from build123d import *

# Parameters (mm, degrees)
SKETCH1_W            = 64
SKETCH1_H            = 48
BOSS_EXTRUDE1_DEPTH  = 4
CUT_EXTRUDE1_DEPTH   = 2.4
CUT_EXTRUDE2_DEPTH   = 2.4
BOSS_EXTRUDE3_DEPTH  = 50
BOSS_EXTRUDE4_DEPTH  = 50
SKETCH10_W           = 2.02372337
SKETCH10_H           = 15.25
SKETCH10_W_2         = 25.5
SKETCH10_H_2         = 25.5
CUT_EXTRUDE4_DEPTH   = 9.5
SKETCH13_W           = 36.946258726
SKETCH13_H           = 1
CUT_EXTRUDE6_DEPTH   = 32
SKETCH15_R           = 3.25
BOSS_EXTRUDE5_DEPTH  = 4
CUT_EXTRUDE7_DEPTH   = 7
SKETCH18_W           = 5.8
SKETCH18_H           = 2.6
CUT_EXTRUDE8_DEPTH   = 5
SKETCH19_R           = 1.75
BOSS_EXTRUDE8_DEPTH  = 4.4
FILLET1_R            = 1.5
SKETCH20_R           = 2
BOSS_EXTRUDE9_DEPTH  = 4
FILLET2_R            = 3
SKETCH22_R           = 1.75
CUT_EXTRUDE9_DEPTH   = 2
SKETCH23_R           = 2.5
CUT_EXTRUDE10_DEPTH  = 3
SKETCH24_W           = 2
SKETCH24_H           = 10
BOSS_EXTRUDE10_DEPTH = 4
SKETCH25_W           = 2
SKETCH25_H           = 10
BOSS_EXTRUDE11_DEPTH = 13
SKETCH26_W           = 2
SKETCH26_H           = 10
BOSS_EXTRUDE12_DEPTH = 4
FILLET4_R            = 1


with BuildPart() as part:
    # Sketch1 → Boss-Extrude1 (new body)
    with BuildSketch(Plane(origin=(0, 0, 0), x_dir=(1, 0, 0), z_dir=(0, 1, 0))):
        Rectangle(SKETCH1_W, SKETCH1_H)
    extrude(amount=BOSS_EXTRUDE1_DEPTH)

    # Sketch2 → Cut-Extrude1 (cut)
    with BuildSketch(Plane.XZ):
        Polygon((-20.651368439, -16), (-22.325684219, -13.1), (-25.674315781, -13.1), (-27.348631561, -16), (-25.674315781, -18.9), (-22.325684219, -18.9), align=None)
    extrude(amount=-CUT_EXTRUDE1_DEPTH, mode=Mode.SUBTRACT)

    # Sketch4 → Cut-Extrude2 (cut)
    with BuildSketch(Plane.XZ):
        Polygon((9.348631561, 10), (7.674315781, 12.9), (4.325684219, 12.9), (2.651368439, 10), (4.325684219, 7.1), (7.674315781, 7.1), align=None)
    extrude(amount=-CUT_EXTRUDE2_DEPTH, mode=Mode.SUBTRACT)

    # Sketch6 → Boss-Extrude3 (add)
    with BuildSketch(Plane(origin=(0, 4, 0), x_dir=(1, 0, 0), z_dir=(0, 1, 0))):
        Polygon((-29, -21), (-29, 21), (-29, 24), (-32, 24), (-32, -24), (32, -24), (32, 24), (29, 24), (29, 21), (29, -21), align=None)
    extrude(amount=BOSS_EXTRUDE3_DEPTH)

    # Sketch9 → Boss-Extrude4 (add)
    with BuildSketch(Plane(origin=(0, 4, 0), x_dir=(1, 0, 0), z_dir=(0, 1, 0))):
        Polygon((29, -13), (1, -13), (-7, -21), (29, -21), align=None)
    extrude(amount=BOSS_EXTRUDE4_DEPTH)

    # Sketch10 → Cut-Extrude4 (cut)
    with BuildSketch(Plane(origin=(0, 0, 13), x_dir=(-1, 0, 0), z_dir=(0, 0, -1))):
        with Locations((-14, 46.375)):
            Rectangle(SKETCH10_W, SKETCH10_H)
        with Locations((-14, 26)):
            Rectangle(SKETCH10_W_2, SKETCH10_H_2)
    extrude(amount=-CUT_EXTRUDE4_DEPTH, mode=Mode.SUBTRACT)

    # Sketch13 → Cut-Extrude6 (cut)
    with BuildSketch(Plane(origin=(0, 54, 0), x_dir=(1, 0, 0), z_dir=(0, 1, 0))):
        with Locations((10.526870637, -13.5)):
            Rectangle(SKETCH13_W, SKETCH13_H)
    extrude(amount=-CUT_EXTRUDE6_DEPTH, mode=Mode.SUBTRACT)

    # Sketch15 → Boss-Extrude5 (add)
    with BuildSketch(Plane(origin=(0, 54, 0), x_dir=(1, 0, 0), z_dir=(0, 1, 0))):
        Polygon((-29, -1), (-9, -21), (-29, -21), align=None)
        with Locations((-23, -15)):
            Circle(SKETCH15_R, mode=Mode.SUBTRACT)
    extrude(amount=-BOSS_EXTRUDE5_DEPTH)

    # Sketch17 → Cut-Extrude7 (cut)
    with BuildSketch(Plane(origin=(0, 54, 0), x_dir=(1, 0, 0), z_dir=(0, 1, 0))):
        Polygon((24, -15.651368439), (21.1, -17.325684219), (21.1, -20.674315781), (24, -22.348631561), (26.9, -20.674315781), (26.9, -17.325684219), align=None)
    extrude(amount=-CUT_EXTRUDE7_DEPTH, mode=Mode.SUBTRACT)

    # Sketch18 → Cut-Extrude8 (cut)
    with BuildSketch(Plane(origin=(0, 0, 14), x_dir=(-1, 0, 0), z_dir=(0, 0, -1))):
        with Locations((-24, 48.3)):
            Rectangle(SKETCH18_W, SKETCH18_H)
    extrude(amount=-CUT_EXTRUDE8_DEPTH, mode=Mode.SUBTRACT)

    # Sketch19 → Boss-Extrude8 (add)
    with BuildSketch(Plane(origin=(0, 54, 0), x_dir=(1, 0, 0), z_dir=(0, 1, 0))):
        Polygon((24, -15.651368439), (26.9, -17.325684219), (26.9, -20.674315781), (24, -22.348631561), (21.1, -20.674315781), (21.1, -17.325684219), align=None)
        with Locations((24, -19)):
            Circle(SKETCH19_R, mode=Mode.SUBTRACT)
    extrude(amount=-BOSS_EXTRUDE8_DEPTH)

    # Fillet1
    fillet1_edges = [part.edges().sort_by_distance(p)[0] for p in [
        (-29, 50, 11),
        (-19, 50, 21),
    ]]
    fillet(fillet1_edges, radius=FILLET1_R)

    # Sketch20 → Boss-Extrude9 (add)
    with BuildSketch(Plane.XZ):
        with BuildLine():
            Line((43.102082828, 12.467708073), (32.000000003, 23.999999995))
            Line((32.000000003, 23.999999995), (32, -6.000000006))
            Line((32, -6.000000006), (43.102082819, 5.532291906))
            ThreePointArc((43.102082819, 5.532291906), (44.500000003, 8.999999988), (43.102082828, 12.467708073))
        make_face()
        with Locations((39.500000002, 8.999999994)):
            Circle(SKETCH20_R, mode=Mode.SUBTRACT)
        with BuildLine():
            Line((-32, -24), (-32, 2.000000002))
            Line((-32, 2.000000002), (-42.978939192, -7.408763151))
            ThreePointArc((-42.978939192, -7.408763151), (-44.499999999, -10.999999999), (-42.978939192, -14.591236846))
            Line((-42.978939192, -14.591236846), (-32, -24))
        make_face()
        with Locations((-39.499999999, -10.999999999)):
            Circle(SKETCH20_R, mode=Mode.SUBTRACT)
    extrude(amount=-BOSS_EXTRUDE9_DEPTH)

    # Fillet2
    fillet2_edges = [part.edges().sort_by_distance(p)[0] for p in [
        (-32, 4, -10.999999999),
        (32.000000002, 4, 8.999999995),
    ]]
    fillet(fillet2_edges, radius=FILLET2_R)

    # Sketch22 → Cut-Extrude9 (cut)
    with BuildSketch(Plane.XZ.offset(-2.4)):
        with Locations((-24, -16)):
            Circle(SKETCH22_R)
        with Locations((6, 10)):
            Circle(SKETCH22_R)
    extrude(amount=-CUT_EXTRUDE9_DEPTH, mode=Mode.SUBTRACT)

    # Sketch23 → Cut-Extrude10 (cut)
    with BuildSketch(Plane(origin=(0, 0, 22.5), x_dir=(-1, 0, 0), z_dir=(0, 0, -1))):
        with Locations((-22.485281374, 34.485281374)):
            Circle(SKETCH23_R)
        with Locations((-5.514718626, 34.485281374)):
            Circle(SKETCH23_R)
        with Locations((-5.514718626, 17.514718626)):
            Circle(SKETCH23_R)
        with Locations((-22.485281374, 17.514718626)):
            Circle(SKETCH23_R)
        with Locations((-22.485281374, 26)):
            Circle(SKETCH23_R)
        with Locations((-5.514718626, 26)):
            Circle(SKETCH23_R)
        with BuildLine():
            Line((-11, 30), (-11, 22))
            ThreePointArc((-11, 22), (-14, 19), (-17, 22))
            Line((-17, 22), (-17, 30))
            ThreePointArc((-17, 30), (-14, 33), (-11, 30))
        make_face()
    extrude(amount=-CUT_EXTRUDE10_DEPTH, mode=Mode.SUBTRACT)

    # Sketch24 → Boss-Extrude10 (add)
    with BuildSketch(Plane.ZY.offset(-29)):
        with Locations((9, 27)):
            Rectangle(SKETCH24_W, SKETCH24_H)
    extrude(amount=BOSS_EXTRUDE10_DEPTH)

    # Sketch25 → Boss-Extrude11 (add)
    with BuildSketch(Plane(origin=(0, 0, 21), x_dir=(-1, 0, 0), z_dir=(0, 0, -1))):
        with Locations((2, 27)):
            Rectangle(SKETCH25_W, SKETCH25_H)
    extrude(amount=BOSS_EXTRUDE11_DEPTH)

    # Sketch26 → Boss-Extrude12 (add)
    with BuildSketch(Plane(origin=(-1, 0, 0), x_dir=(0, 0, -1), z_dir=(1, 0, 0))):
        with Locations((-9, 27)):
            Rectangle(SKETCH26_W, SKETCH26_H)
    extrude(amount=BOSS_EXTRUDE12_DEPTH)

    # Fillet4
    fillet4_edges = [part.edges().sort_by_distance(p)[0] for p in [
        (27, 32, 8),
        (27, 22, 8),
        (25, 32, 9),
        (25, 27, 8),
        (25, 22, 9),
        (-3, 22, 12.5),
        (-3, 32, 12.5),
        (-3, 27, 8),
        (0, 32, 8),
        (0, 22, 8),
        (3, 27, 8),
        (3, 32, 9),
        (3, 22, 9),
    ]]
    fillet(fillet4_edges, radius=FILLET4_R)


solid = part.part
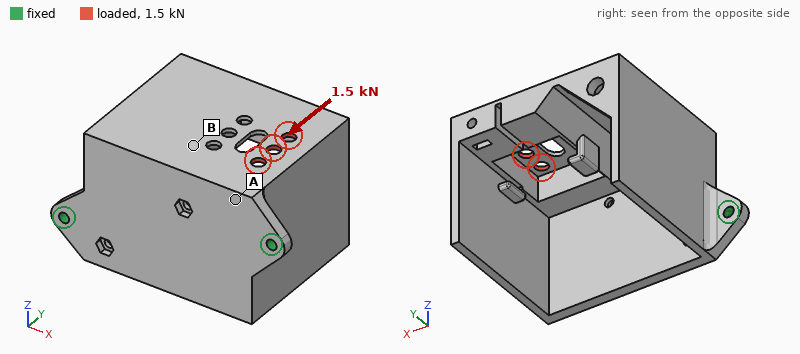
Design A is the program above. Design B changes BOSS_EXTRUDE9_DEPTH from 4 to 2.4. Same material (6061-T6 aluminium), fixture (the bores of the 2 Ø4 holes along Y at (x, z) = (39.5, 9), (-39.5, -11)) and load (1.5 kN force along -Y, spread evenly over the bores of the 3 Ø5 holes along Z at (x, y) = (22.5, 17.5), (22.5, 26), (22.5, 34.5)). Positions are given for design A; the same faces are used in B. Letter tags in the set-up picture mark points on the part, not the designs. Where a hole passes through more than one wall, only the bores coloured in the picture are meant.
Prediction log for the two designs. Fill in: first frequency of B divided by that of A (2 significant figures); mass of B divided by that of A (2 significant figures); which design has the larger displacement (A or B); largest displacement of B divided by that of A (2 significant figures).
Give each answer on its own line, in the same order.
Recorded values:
0.57
0.99
B
3.0
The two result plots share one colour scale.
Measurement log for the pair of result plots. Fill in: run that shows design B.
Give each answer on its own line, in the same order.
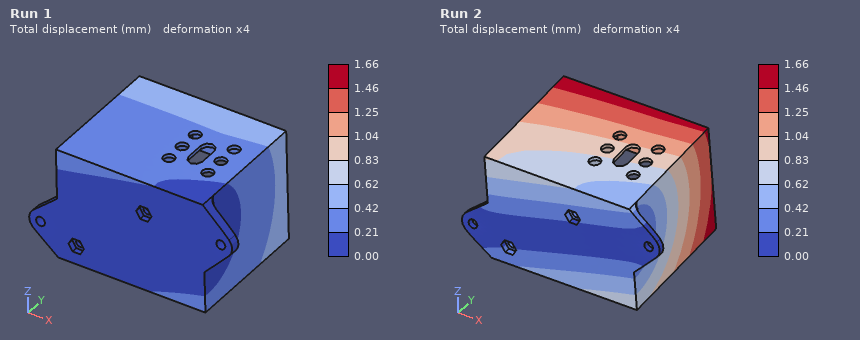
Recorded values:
Run 2
